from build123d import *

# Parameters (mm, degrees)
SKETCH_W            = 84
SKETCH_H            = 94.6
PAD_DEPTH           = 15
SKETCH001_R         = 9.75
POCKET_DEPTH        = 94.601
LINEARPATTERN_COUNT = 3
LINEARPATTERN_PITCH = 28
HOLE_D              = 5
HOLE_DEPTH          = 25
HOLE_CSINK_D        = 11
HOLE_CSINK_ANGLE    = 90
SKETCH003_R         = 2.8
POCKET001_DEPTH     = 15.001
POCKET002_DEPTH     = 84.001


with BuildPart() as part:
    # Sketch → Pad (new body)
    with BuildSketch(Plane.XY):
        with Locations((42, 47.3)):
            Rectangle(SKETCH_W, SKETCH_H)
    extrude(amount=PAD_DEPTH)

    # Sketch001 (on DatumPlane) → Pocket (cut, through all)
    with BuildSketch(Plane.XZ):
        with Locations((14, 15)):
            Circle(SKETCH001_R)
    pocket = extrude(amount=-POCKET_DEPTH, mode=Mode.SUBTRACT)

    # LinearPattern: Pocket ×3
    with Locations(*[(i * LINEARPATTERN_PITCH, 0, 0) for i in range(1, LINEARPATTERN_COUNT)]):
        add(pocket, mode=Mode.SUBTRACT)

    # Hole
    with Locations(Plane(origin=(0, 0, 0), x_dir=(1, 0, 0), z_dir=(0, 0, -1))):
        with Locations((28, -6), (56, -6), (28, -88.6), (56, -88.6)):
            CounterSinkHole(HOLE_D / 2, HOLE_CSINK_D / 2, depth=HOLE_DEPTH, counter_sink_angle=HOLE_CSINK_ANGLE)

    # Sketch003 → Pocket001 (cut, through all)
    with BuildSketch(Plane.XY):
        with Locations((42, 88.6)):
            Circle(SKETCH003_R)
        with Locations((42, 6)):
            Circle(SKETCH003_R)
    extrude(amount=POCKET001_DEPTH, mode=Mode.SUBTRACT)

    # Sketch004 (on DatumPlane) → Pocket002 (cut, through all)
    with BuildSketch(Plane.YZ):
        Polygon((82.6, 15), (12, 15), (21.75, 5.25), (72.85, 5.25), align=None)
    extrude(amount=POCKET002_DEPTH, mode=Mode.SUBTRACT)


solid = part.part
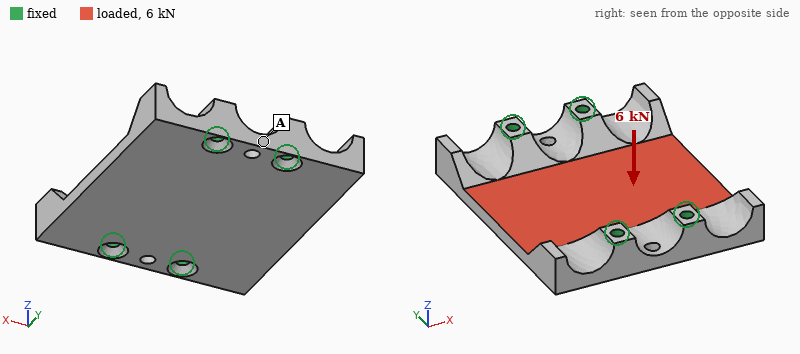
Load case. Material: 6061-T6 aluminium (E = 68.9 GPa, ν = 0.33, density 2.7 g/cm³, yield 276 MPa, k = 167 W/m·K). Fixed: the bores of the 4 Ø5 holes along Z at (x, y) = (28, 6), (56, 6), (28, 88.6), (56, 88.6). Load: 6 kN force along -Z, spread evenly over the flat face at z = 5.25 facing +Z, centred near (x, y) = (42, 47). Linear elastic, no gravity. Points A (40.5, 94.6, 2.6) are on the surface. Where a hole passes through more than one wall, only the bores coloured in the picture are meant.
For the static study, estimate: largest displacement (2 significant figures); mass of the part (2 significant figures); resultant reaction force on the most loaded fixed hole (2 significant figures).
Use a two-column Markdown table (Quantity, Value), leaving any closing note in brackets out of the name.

| Quantity | Value |
|---|---|
| largest displacement | 0.15 mm |
| mass of the part | 140 g |
| resultant reaction force on the most loaded fixed hole | 2.2 kN |
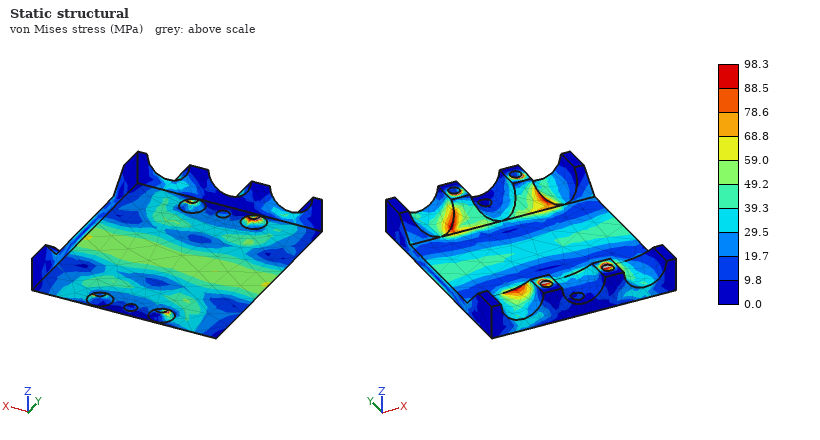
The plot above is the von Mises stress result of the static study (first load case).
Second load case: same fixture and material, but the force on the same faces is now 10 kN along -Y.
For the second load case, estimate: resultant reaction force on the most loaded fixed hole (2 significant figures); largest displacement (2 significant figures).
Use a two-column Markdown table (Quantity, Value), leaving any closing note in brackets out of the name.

| Quantity | Value |
|---|---|
| resultant reaction force on the most loaded fixed hole | 2.5 kN |
| largest displacement | 16 µm |
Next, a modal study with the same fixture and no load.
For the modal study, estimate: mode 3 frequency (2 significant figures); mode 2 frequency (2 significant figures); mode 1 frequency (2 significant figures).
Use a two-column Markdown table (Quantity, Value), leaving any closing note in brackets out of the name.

| Quantity | Value |
|---|---|
| mode 3 frequency | 6400 Hz |
| mode 2 frequency | 4700 Hz |
| mode 1 frequency | 4500 Hz |
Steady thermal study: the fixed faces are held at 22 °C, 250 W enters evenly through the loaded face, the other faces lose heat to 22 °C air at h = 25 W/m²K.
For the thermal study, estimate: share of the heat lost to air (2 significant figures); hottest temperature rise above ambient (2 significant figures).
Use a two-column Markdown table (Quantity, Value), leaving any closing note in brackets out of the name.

| Quantity | Value |
|---|---|
| share of the heat lost to air | 3.8 % |
| hottest temperature rise above ambient | 51 K |
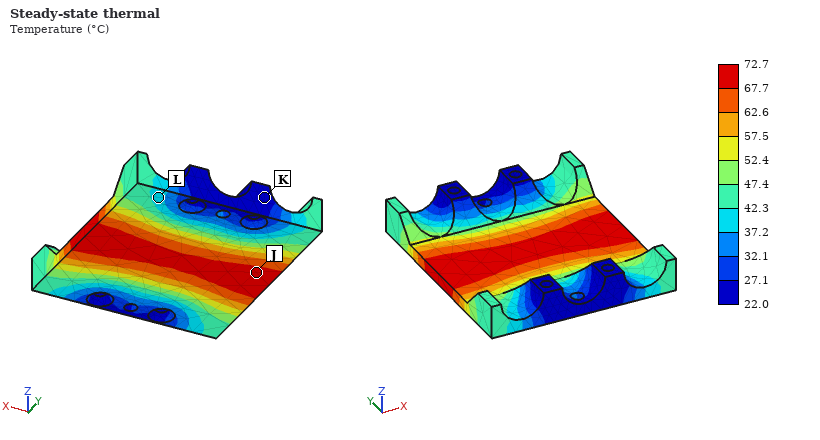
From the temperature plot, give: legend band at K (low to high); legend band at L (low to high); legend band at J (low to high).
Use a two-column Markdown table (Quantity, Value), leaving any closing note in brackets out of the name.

| Quantity | Value |
|---|---|
| legend band at K | 22.0 to 27.1 °C |
| legend band at L | 37.2 to 42.3 °C |
| legend band at J | 67.7 to 72.7 °C |
